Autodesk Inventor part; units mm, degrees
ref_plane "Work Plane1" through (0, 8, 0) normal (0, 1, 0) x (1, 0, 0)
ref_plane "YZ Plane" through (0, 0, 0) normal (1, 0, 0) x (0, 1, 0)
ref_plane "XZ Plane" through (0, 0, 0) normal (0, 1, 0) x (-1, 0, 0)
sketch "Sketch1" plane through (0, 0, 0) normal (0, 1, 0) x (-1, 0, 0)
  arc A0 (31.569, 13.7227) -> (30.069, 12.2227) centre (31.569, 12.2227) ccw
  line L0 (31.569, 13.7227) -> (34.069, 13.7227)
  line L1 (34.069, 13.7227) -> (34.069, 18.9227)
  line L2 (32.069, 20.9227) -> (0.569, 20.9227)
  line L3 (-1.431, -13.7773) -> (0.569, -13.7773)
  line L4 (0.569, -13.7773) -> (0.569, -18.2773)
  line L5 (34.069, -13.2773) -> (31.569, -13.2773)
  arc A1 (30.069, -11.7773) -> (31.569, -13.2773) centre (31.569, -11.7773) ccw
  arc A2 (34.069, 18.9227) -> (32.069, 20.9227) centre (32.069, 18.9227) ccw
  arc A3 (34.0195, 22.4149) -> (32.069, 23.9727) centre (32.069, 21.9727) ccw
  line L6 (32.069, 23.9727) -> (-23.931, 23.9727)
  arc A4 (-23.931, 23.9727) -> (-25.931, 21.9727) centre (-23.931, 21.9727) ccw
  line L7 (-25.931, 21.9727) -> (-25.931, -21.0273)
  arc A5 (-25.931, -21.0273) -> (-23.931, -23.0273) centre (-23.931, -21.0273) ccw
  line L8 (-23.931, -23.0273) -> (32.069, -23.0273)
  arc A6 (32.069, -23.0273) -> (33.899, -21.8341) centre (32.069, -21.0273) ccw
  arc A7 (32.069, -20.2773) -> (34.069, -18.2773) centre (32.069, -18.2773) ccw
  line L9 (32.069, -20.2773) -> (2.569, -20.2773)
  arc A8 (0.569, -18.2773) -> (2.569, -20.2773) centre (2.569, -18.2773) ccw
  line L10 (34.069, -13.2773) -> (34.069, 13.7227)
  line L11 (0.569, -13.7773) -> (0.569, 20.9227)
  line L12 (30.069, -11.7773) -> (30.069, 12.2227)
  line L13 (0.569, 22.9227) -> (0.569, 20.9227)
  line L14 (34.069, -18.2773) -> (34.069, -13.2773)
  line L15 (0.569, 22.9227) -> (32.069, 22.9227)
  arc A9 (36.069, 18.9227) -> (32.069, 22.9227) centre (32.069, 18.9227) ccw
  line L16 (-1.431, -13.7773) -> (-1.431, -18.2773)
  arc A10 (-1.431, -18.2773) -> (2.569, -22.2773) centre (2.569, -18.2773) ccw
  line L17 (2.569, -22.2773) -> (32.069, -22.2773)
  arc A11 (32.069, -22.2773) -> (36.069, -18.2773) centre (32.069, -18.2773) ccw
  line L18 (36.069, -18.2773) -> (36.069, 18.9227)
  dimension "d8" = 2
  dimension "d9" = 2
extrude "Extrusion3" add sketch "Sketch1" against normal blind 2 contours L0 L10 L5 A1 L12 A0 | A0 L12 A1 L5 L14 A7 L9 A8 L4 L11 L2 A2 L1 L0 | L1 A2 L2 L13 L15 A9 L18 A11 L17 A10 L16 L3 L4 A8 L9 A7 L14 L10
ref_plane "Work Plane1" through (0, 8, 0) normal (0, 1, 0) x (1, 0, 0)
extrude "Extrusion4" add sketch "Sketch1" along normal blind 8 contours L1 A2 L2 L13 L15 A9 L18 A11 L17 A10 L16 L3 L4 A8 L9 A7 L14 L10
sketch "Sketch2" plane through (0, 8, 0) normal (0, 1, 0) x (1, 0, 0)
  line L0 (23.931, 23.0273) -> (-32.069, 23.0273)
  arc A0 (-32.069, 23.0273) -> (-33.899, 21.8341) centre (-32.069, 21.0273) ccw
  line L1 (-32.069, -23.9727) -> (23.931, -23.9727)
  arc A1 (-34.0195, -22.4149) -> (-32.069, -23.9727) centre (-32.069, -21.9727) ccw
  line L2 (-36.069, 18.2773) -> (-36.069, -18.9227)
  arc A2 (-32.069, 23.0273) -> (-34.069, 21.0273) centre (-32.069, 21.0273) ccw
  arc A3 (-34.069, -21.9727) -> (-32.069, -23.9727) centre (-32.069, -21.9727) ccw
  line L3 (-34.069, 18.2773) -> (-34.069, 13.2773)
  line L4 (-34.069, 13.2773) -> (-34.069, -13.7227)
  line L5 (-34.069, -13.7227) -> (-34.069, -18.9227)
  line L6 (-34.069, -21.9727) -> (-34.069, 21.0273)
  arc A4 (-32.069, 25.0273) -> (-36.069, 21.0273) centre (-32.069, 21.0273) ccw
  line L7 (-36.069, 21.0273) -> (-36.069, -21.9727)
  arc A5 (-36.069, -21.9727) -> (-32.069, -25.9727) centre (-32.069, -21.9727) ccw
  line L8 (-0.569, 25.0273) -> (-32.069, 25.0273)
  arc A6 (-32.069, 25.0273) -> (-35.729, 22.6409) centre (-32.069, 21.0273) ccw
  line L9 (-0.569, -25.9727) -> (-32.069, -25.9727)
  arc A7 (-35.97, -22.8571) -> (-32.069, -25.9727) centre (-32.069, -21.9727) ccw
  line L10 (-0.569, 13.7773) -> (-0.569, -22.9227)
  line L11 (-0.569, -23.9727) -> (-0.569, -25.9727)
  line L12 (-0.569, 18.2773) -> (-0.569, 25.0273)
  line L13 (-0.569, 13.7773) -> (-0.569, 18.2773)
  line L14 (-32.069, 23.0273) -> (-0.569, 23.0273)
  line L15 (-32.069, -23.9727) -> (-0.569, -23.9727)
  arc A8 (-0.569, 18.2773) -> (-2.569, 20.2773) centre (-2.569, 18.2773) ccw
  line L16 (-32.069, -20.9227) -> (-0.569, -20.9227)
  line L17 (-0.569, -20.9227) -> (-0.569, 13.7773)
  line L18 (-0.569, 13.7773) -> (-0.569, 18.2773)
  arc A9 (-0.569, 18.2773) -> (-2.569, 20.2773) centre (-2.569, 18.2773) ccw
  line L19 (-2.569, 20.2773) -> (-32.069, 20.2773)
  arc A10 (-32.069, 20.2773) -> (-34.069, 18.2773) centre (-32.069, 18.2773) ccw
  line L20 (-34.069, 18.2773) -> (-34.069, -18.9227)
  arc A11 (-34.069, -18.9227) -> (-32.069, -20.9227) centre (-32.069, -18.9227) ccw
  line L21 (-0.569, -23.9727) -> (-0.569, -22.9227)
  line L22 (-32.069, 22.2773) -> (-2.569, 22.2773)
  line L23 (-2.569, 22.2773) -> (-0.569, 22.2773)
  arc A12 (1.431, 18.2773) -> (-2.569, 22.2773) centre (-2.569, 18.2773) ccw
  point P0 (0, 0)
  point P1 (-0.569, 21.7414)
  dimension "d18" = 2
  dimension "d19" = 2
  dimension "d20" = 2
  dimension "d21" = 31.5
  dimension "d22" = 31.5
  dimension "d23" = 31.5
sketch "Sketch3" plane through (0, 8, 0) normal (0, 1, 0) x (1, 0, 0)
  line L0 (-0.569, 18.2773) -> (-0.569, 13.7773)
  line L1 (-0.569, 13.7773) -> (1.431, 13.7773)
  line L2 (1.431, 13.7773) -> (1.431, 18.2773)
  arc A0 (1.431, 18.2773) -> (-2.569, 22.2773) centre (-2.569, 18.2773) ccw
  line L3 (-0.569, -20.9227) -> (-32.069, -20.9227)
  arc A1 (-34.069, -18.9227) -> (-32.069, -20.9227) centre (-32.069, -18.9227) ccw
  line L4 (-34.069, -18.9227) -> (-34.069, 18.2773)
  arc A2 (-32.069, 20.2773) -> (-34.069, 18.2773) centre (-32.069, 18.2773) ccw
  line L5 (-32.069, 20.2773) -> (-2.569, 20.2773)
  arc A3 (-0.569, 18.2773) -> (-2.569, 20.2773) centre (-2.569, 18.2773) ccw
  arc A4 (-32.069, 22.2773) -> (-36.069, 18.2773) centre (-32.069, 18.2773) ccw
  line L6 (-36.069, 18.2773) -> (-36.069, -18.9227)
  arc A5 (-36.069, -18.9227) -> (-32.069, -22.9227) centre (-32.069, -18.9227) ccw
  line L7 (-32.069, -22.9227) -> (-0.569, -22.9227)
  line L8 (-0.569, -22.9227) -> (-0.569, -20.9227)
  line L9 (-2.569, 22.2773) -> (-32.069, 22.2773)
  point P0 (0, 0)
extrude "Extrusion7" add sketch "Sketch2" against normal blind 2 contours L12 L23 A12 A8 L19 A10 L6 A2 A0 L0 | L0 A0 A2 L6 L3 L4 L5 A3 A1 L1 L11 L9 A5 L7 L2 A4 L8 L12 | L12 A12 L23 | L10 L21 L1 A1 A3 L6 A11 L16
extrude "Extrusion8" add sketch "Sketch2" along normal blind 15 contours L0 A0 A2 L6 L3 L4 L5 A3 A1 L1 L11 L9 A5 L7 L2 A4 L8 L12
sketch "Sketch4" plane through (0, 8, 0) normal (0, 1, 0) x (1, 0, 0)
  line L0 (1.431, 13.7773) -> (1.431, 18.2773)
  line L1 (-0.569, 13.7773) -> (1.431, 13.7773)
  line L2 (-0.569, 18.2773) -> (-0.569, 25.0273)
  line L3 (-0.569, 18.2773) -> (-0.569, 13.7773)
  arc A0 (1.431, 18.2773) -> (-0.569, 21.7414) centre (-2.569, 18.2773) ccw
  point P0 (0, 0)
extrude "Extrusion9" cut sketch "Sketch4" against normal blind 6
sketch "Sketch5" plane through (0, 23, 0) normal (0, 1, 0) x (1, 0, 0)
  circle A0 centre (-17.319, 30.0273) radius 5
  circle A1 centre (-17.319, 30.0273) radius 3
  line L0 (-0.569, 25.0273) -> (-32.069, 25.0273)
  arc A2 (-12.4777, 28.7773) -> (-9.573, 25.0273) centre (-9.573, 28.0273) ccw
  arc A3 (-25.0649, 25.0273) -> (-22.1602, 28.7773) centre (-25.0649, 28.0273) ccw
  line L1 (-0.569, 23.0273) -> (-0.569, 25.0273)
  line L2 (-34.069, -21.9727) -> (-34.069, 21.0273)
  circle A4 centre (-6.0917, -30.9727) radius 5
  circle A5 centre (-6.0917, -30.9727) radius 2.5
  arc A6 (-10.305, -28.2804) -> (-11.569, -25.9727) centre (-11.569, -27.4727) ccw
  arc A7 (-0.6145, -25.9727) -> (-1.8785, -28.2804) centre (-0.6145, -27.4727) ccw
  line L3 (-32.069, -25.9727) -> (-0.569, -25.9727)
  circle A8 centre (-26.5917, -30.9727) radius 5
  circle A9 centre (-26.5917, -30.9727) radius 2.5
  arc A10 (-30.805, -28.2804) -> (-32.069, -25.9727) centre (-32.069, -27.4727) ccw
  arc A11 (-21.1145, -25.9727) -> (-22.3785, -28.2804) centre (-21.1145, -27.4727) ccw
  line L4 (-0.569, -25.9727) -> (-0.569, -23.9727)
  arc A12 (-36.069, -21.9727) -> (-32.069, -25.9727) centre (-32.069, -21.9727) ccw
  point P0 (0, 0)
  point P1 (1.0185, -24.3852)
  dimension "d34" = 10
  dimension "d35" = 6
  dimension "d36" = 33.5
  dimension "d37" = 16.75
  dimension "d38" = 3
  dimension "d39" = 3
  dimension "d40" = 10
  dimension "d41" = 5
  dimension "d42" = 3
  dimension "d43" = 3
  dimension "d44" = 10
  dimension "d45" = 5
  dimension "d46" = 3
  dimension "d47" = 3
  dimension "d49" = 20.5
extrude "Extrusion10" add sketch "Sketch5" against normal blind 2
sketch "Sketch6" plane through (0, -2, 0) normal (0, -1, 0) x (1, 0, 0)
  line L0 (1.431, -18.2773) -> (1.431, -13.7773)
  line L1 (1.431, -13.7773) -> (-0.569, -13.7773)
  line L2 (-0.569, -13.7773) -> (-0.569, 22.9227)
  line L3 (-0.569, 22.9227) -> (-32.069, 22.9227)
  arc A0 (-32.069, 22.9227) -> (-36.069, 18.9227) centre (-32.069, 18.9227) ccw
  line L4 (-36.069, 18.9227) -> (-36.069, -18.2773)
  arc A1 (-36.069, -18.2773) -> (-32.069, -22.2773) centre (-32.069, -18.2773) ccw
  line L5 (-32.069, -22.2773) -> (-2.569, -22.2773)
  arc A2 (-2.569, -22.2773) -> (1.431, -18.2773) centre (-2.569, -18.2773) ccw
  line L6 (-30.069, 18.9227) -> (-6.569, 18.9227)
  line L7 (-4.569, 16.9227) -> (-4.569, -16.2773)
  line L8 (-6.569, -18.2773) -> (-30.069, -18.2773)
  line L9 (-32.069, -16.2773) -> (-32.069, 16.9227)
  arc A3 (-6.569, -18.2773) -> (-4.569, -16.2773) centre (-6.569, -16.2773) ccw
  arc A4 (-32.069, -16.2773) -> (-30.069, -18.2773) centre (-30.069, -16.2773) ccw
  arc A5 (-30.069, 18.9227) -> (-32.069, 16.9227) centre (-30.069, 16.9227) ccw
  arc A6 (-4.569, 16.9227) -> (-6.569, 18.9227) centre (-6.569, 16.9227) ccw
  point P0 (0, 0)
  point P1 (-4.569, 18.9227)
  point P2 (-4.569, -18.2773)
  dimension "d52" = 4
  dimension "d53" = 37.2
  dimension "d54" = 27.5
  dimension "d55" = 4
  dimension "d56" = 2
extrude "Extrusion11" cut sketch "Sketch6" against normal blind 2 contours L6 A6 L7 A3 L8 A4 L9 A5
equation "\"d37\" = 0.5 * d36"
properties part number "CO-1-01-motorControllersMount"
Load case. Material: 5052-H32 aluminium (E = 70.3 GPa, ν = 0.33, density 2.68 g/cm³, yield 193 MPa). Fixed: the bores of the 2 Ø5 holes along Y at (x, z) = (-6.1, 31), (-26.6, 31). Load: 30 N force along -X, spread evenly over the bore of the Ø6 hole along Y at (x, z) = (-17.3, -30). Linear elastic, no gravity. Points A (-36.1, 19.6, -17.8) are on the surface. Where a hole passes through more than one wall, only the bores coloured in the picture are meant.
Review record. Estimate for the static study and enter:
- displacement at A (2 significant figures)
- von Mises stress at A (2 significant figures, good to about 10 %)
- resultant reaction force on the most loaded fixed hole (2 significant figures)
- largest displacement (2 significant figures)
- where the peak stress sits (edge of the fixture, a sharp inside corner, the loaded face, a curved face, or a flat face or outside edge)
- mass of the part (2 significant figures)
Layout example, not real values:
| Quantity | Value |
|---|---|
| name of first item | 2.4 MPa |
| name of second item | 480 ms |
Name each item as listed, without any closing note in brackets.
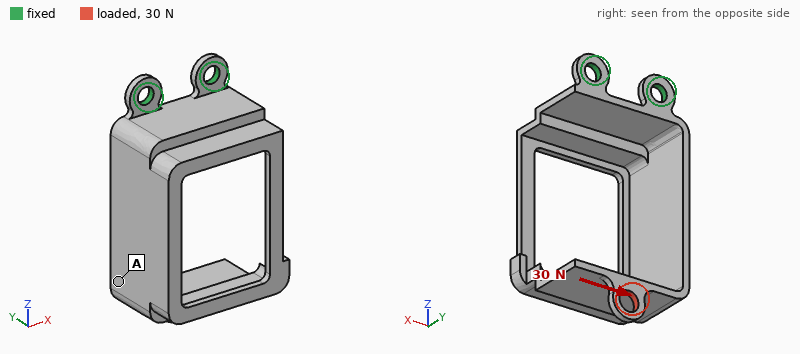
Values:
| Quantity | Value |
|---|---|
| displacement at A | 0.57 mm |
| von Mises stress at A | 21 MPa |
| resultant reaction force on the most loaded fixed hole | 59 N |
| largest displacement | 0.76 mm |
| where the peak stress sits | a curved face |
| mass of the part | 19 g |
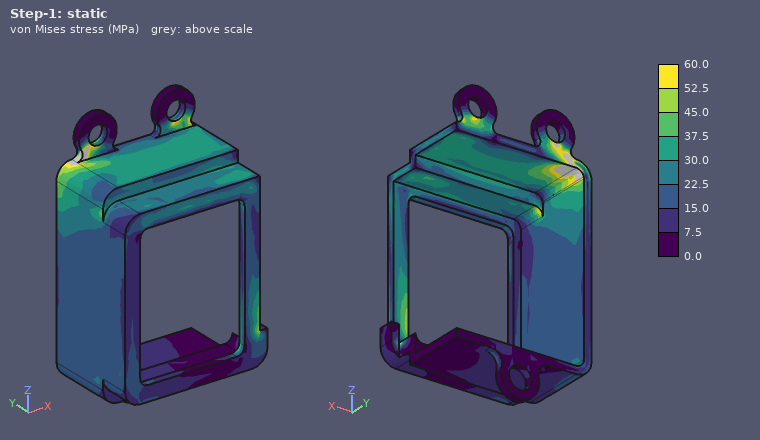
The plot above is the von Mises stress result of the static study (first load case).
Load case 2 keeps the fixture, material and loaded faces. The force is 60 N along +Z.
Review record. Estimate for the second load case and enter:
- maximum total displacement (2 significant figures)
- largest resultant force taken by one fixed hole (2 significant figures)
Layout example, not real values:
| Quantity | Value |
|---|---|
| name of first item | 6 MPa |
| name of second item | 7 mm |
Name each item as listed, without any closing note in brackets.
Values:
| Quantity | Value |
|---|---|
| maximum total displacement | 0.54 mm |
| largest resultant force taken by one fixed hole | 33 N |
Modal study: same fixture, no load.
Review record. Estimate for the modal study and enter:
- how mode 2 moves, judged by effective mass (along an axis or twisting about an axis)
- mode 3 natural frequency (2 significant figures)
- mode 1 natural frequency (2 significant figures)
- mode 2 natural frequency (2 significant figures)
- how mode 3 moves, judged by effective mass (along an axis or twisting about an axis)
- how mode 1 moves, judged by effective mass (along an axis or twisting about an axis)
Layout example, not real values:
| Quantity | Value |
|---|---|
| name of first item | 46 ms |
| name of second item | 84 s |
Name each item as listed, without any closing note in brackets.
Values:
| Quantity | Value |
|---|---|
| how mode 2 moves, judged by effective mass | along X |
| mode 3 natural frequency | 1200 Hz |
| mode 1 natural frequency | 300 Hz |
| mode 2 natural frequency | 480 Hz |
| how mode 3 moves, judged by effective mass | along Z |
| how mode 1 moves, judged by effective mass | along Y |
